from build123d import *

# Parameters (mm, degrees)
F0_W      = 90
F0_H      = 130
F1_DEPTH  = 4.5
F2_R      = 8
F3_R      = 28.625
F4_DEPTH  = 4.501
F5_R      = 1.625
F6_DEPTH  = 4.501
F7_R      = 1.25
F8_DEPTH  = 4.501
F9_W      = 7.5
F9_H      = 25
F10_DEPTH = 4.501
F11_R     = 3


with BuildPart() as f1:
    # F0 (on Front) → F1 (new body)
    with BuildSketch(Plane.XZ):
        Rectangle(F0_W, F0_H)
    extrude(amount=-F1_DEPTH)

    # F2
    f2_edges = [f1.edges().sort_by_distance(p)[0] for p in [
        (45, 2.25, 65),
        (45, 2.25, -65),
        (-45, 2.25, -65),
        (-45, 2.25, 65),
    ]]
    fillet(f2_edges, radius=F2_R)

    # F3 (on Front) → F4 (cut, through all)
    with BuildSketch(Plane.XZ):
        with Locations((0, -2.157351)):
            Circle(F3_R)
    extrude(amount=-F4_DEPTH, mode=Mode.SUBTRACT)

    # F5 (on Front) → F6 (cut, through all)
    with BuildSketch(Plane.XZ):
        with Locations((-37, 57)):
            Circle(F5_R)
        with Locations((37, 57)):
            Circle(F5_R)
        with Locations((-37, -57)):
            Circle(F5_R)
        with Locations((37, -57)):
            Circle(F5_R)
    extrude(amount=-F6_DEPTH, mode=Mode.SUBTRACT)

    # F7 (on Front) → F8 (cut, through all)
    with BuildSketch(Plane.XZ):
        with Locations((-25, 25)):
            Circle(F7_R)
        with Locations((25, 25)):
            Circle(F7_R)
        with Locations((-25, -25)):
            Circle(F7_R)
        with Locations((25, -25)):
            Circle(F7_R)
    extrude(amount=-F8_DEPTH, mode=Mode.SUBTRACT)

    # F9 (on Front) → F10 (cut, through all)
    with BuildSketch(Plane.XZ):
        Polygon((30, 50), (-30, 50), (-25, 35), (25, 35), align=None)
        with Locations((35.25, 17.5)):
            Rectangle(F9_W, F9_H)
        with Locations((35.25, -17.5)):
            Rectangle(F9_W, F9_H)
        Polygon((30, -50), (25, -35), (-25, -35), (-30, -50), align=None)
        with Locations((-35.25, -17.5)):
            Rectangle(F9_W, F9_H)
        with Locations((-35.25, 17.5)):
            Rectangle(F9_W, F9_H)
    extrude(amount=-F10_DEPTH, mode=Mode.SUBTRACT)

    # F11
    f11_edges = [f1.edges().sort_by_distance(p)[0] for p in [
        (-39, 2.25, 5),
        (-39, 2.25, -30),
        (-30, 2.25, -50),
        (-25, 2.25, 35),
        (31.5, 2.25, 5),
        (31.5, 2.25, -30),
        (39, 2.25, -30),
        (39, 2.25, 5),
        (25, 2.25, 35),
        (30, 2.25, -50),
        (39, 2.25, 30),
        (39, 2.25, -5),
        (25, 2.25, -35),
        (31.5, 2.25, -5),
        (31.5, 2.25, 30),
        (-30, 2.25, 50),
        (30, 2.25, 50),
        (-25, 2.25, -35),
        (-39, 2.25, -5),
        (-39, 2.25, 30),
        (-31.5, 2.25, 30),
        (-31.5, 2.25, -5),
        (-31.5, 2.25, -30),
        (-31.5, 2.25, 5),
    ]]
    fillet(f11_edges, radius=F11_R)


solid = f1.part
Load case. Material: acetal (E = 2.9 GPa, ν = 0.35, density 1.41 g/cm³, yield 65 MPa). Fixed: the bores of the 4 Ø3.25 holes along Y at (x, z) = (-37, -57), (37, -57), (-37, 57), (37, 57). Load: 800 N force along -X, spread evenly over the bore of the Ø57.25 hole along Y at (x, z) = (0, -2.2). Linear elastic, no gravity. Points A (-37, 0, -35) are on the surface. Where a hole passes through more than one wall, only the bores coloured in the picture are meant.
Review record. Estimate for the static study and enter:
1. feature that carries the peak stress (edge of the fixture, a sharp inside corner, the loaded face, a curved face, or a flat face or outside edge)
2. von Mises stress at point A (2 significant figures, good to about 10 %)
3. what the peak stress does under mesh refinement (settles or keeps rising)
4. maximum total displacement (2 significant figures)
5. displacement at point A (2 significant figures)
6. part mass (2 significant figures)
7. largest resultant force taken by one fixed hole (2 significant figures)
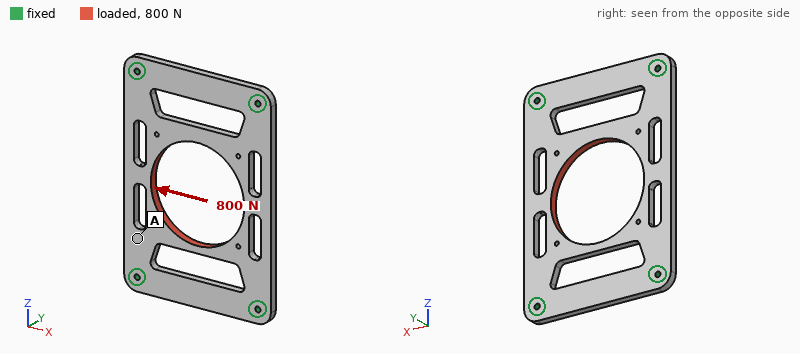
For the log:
edge of the fixture
5.7 MPa
keeps rising
0.56 mm
0.20 mm
42 g
250 N
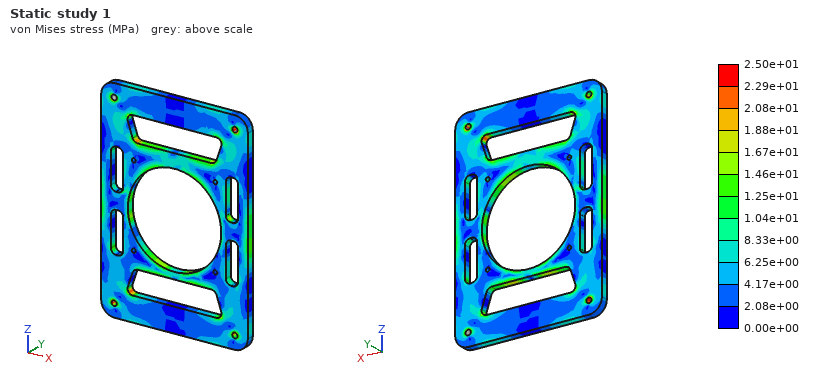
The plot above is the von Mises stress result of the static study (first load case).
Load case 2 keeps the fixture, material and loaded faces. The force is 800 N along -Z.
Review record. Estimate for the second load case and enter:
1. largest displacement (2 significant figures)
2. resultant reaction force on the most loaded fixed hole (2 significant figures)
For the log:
0.33 mm
210 N
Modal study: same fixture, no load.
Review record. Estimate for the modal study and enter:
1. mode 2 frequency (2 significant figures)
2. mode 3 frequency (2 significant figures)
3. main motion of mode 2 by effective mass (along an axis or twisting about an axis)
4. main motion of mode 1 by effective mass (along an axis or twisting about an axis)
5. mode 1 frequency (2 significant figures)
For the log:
580 Hz
870 Hz
twisting about Z
along Y
460 Hz
